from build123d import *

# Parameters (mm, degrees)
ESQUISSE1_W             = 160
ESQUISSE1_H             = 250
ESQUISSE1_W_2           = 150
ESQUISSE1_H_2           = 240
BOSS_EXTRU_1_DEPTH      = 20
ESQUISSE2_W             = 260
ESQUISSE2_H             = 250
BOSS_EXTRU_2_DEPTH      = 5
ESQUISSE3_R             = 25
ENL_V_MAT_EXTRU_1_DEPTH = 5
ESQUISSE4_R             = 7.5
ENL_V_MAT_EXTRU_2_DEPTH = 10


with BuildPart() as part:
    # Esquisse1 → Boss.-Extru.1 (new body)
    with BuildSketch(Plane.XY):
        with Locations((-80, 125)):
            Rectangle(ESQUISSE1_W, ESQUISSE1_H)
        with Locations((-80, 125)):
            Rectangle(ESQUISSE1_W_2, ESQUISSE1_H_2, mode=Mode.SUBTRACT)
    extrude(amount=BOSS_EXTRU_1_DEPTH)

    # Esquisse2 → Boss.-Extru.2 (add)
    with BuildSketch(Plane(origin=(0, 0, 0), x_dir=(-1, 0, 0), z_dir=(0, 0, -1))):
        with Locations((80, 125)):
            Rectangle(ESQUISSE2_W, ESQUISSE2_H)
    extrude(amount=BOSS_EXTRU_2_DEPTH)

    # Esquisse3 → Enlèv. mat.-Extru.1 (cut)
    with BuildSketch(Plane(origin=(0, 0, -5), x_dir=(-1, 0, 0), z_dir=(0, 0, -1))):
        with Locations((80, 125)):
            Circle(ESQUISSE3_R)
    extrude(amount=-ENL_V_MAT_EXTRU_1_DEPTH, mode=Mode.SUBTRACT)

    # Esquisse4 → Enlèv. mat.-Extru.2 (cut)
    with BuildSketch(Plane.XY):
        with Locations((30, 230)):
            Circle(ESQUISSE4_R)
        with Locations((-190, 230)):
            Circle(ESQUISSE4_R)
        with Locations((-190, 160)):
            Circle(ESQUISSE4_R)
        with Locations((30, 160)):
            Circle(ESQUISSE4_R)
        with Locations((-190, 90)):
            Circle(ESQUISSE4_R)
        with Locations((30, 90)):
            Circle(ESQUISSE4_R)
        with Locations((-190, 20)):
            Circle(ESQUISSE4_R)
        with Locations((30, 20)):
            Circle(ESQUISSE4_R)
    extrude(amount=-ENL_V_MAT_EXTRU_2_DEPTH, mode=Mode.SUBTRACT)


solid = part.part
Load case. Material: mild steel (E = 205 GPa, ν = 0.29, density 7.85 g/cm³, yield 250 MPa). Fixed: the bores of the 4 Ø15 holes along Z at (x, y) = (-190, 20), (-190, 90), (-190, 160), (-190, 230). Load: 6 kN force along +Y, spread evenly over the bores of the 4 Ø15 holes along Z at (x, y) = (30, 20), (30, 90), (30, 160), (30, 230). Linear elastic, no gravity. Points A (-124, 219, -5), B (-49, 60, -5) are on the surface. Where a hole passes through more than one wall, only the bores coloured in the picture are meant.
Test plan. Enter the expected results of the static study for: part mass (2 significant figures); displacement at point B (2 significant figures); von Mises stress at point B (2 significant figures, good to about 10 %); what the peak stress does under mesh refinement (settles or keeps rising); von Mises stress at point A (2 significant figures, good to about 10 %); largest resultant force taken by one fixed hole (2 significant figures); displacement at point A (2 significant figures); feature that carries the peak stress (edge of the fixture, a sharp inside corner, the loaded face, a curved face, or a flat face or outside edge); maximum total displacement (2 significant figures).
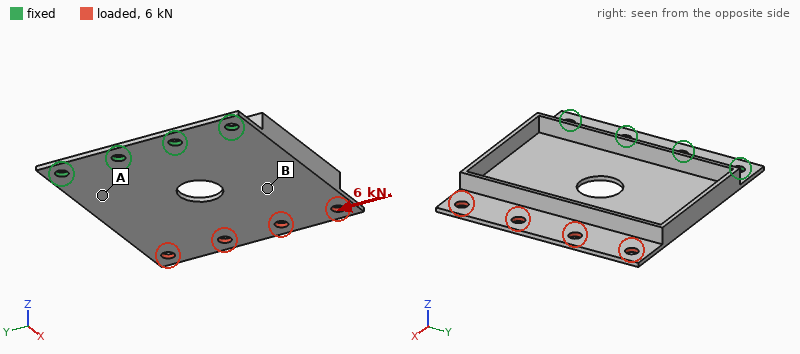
3.0 kg
21 µm
9.1 MPa
keeps rising
17 MPa
5.8 kN
11 µm
edge of the fixture
45 µm
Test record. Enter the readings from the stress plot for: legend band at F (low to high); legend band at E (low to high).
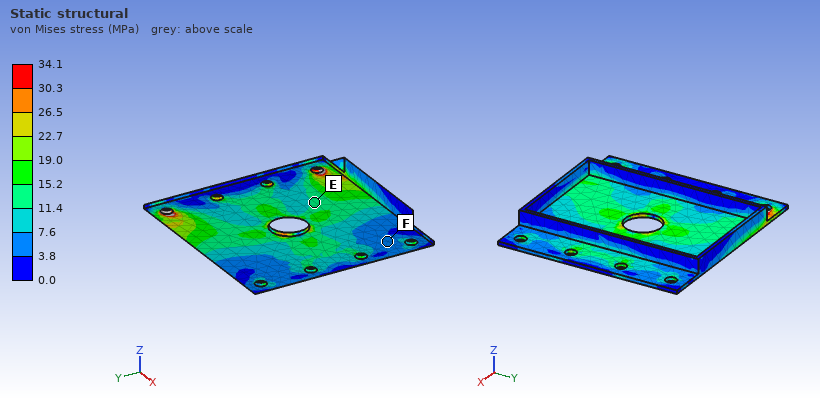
3.8 to 7.6 MPa
11.4 to 15.2 MPa
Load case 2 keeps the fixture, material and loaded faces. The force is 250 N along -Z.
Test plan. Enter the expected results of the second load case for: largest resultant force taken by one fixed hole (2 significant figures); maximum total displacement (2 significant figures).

360 N
0.96 mm
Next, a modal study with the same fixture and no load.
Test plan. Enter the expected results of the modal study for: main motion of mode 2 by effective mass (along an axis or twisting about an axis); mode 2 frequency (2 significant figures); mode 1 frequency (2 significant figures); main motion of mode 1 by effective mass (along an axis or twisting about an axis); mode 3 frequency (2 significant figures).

twisting about X
180 Hz
88 Hz
along Z
690 Hz
